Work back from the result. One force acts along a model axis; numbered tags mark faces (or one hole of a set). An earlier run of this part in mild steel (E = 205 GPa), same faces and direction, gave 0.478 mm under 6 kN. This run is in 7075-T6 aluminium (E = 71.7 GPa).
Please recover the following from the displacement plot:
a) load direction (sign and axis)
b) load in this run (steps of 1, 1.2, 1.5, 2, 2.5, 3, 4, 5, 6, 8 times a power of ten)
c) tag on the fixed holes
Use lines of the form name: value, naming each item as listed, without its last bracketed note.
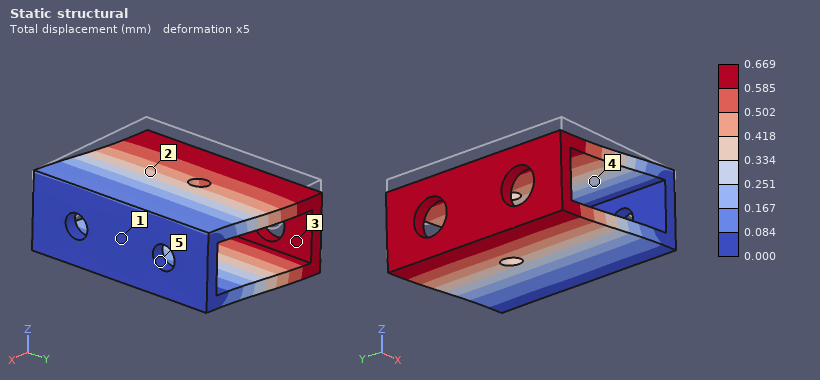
load direction: -Z
load in this run: 3 kN
tag on the fixed holes: 5
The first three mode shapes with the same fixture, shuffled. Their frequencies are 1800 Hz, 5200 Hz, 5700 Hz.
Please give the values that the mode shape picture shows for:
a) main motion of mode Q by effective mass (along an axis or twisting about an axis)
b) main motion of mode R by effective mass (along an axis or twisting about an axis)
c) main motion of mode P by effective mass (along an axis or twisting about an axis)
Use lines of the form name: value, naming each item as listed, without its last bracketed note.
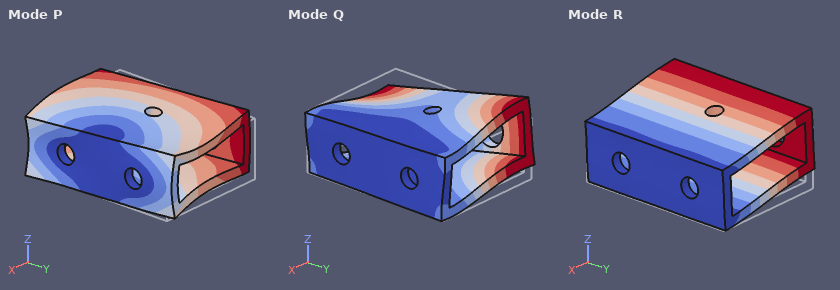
main motion of mode Q by effective mass: twisting about X
main motion of mode R by effective mass: along Z
main motion of mode P by effective mass: along Y
